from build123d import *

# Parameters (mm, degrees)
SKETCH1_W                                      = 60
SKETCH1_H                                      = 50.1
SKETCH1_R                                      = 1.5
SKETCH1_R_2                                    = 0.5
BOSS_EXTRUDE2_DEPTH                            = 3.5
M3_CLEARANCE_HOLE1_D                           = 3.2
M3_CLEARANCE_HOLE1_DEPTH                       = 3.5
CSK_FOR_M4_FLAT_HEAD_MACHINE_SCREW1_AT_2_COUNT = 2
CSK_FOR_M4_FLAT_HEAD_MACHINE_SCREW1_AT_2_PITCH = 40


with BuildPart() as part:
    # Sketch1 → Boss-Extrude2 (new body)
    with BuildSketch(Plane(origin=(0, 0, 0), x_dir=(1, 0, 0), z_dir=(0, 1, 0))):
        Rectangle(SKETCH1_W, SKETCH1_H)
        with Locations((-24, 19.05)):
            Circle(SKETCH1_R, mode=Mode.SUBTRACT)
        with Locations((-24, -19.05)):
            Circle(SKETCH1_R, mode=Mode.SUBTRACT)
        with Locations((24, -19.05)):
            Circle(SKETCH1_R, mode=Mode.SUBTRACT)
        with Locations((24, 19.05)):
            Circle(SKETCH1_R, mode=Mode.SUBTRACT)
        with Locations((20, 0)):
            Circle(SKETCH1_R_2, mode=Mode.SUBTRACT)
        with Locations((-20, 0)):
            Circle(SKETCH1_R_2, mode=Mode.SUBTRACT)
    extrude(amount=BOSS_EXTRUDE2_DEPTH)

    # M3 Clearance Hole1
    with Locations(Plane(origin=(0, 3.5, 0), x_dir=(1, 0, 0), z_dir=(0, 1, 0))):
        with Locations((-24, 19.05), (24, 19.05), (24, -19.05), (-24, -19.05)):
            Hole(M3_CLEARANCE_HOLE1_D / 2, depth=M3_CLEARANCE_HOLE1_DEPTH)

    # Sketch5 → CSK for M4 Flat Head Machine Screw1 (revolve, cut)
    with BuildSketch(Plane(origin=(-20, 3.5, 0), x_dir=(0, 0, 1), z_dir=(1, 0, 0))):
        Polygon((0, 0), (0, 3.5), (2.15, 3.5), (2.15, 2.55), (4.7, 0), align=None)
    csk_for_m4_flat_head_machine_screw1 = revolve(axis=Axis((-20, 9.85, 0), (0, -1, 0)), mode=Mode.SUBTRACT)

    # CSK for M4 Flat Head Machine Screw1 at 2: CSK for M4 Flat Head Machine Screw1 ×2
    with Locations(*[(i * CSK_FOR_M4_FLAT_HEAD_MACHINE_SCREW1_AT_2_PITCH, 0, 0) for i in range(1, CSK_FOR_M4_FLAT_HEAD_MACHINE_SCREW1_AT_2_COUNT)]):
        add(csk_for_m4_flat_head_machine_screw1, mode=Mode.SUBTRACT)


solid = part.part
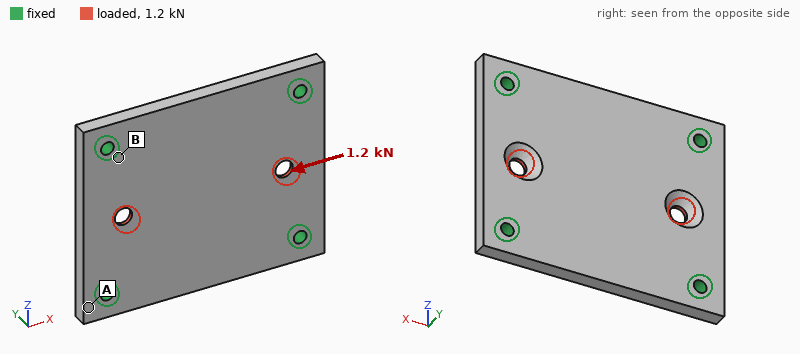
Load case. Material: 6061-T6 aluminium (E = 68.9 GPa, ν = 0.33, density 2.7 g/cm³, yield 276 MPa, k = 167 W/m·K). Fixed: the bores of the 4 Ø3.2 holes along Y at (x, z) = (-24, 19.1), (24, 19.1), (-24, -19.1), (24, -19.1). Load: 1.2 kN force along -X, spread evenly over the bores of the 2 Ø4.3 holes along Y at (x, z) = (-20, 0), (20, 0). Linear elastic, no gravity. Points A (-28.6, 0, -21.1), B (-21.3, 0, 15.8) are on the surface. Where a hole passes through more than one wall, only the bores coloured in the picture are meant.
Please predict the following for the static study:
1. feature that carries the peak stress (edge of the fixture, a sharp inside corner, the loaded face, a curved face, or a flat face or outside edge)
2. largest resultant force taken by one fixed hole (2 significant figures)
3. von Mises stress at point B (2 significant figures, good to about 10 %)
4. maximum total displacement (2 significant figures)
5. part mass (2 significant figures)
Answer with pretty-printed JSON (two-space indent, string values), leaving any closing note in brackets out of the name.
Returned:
{
  "feature that carries the peak stress": "the loaded face",
  "largest resultant force taken by one fixed hole": "320 N",
  "von Mises stress at point B": "11 MPa",
  "maximum total displacement": "6.4 µm",
  "part mass": "27 g"
}
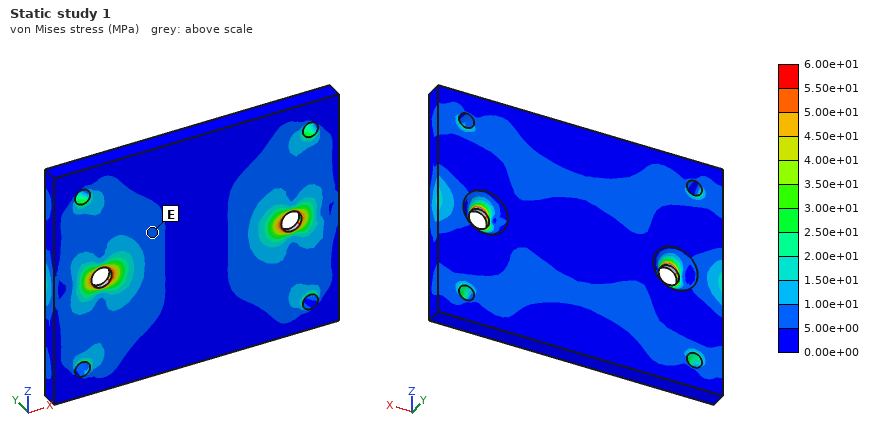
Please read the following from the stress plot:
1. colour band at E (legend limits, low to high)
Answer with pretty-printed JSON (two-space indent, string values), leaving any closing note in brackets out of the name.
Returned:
{
  "colour band at E": "5.00e+00 to 1.00e+01 MPa"
}
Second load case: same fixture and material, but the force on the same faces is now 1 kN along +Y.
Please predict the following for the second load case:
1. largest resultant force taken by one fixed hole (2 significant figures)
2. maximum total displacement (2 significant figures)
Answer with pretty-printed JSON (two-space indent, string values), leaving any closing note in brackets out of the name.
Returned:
{
  "largest resultant force taken by one fixed hole": "260 N",
  "maximum total displacement": "48 µm"
}
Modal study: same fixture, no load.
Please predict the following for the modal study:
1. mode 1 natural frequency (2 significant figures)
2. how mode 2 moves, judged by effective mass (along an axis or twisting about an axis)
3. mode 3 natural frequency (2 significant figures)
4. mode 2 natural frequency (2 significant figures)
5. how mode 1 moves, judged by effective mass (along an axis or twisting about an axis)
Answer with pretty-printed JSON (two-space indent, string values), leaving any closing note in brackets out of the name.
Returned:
{
  "mode 1 natural frequency": "6200 Hz",
  "how mode 2 moves, judged by effective mass": "twisting about X",
  "mode 3 natural frequency": "11 kHz",
  "mode 2 natural frequency": "9000 Hz",
  "how mode 1 moves, judged by effective mass": "along Y"
}
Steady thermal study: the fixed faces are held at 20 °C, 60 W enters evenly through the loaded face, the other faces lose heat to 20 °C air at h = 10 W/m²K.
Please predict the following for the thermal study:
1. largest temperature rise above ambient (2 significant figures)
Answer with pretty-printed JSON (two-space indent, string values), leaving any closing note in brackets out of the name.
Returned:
{
  "largest temperature rise above ambient": "40 K"
}
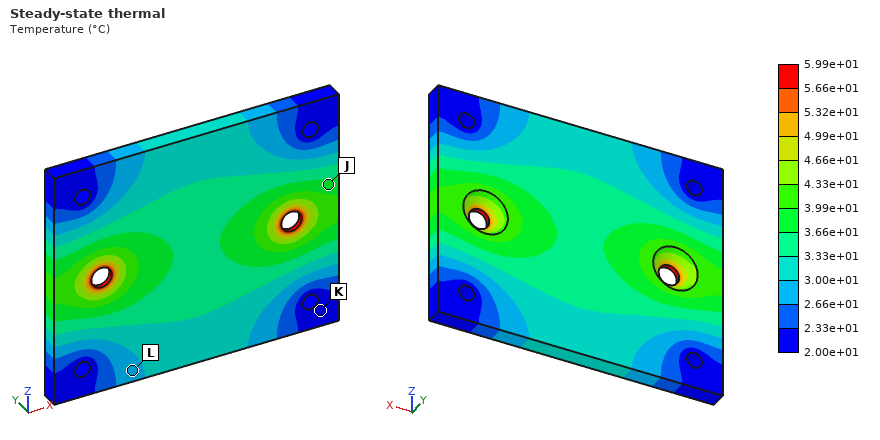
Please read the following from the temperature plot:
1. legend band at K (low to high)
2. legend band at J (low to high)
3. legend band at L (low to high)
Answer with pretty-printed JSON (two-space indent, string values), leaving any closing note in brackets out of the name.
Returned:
{
  "legend band at K": "2.00e+01 to 2.33e+01 °C",
  "legend band at J": "3.66e+01 to 3.99e+01 °C",
  "legend band at L": "2.66e+01 to 3.00e+01 °C"
}
